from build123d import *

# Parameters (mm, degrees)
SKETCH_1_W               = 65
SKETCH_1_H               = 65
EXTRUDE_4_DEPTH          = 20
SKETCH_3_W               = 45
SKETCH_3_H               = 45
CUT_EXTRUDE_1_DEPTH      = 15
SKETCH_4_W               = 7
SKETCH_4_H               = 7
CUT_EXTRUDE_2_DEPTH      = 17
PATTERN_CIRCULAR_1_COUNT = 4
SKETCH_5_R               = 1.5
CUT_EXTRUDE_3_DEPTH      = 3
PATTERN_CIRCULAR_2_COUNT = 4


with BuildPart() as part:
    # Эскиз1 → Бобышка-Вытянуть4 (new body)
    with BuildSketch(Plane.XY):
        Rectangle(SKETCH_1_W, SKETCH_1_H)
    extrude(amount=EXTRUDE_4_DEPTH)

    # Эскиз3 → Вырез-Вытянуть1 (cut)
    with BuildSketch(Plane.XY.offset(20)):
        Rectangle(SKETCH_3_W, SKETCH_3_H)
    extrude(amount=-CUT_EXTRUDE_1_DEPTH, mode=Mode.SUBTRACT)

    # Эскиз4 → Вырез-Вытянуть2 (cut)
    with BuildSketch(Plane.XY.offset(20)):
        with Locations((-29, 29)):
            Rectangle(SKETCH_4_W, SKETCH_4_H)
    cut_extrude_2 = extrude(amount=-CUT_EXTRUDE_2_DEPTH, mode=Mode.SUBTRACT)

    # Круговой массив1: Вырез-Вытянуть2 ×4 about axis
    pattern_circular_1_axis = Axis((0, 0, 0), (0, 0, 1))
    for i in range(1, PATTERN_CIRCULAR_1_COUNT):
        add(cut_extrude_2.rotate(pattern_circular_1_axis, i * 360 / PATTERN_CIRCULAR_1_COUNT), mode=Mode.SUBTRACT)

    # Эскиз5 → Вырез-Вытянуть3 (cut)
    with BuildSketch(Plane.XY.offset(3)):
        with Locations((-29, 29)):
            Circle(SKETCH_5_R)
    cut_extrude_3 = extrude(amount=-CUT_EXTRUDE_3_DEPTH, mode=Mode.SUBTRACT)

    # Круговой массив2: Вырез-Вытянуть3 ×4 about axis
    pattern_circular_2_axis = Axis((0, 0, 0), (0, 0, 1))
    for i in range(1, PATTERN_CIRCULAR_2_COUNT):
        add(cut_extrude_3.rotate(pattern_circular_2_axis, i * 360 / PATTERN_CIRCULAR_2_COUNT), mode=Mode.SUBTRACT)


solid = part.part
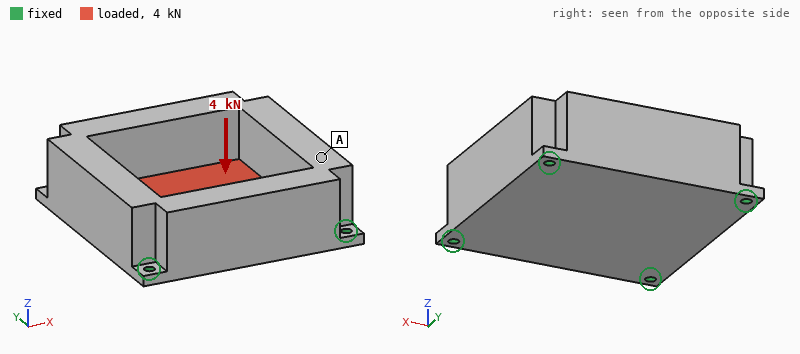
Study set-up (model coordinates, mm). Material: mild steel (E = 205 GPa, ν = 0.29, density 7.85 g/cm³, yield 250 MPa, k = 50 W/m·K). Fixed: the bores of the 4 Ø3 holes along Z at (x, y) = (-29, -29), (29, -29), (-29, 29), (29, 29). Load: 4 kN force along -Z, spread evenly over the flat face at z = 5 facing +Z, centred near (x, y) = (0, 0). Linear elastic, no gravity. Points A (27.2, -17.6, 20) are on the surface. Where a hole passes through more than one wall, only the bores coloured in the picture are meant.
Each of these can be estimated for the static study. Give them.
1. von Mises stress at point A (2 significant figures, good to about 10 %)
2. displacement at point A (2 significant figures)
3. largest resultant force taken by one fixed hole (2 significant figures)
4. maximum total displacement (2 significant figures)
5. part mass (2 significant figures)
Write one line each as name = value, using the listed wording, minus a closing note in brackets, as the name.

von Mises stress at point A = 12 MPa
displacement at point A = 4.4 µm
largest resultant force taken by one fixed hole = 1.2 kN
maximum total displacement = 15 µm
part mass = 400 g
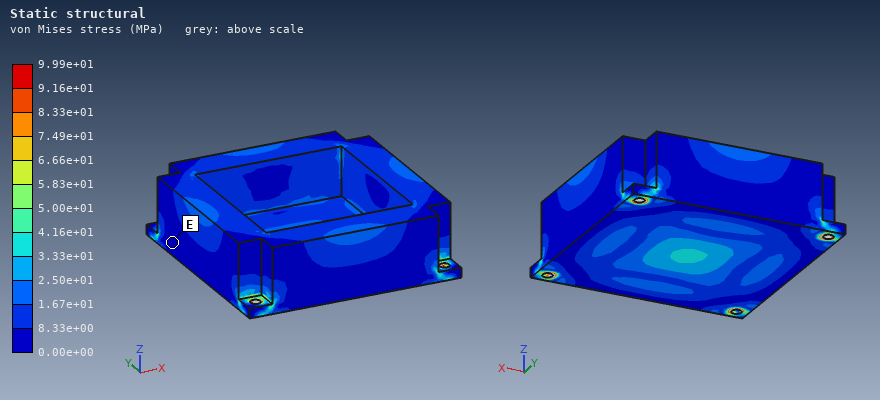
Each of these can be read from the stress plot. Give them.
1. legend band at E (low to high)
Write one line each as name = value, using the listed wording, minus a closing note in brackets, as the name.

legend band at E = 0.00e+00 to 8.33e+00 MPa
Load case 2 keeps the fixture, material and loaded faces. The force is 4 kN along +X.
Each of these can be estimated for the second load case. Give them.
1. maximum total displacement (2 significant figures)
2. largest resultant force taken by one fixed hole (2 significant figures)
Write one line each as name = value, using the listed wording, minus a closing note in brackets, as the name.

maximum total displacement = 2.9 µm
largest resultant force taken by one fixed hole = 1.1 kN
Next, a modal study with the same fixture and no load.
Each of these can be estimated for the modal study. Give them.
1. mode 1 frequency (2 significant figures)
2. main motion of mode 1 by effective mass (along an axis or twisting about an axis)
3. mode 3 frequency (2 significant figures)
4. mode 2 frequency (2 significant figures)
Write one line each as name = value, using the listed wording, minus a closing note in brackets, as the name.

mode 1 frequency = 7700 Hz
main motion of mode 1 by effective mass = along Z
mode 3 frequency = 10000 Hz
mode 2 frequency = 10000 Hz
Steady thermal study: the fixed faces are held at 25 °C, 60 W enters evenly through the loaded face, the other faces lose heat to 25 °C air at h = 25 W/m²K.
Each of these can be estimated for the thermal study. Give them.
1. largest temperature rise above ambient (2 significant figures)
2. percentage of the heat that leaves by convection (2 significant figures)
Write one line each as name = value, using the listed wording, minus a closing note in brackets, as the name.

largest temperature rise above ambient = 62 K
percentage of the heat that leaves by convection = 23 %
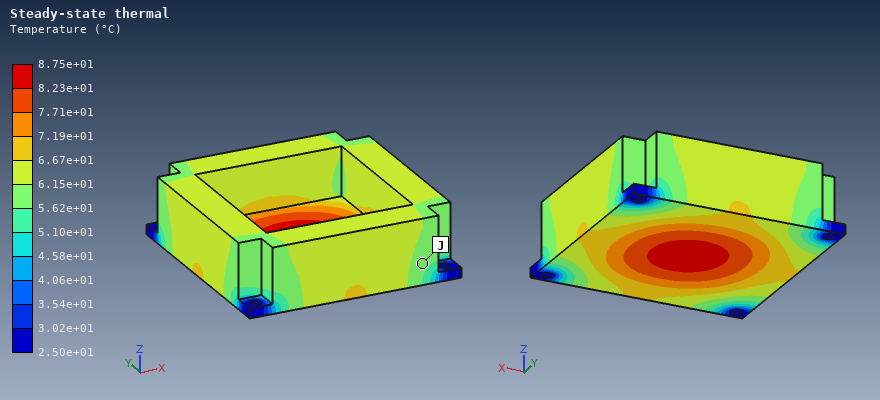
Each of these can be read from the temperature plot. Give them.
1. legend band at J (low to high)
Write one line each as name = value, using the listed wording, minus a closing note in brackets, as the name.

legend band at J = 5.62e+01 to 6.15e+01 °C
